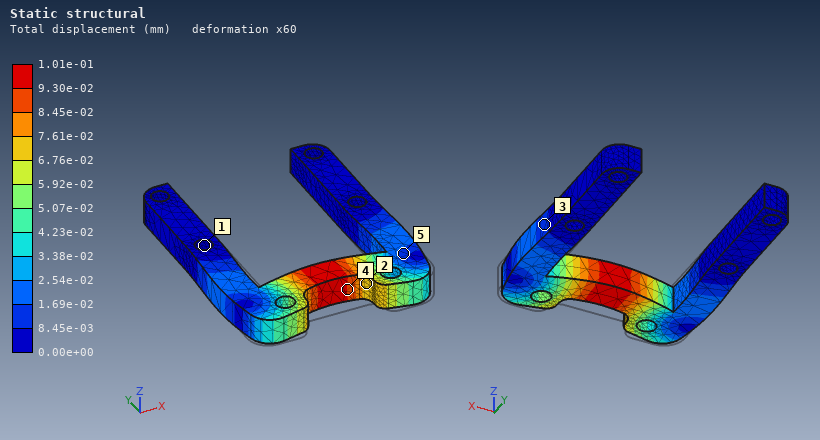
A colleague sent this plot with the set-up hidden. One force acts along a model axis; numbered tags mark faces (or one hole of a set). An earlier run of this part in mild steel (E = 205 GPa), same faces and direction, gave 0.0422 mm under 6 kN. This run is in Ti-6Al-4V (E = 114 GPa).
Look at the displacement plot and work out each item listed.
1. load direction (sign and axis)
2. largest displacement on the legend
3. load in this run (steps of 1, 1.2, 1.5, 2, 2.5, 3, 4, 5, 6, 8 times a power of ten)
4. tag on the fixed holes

+Y
1.01e-01 mm
8 kN
1
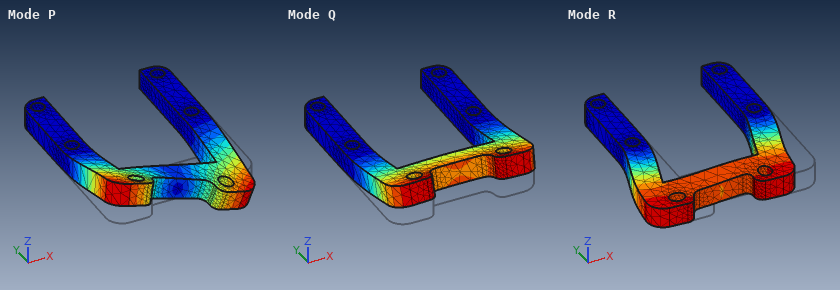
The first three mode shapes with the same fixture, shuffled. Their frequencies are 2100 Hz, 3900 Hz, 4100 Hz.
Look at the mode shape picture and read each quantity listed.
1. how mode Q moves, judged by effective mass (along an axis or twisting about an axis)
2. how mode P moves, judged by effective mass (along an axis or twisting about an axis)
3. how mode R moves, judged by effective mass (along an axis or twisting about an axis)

along Z
twisting about Y
along X
